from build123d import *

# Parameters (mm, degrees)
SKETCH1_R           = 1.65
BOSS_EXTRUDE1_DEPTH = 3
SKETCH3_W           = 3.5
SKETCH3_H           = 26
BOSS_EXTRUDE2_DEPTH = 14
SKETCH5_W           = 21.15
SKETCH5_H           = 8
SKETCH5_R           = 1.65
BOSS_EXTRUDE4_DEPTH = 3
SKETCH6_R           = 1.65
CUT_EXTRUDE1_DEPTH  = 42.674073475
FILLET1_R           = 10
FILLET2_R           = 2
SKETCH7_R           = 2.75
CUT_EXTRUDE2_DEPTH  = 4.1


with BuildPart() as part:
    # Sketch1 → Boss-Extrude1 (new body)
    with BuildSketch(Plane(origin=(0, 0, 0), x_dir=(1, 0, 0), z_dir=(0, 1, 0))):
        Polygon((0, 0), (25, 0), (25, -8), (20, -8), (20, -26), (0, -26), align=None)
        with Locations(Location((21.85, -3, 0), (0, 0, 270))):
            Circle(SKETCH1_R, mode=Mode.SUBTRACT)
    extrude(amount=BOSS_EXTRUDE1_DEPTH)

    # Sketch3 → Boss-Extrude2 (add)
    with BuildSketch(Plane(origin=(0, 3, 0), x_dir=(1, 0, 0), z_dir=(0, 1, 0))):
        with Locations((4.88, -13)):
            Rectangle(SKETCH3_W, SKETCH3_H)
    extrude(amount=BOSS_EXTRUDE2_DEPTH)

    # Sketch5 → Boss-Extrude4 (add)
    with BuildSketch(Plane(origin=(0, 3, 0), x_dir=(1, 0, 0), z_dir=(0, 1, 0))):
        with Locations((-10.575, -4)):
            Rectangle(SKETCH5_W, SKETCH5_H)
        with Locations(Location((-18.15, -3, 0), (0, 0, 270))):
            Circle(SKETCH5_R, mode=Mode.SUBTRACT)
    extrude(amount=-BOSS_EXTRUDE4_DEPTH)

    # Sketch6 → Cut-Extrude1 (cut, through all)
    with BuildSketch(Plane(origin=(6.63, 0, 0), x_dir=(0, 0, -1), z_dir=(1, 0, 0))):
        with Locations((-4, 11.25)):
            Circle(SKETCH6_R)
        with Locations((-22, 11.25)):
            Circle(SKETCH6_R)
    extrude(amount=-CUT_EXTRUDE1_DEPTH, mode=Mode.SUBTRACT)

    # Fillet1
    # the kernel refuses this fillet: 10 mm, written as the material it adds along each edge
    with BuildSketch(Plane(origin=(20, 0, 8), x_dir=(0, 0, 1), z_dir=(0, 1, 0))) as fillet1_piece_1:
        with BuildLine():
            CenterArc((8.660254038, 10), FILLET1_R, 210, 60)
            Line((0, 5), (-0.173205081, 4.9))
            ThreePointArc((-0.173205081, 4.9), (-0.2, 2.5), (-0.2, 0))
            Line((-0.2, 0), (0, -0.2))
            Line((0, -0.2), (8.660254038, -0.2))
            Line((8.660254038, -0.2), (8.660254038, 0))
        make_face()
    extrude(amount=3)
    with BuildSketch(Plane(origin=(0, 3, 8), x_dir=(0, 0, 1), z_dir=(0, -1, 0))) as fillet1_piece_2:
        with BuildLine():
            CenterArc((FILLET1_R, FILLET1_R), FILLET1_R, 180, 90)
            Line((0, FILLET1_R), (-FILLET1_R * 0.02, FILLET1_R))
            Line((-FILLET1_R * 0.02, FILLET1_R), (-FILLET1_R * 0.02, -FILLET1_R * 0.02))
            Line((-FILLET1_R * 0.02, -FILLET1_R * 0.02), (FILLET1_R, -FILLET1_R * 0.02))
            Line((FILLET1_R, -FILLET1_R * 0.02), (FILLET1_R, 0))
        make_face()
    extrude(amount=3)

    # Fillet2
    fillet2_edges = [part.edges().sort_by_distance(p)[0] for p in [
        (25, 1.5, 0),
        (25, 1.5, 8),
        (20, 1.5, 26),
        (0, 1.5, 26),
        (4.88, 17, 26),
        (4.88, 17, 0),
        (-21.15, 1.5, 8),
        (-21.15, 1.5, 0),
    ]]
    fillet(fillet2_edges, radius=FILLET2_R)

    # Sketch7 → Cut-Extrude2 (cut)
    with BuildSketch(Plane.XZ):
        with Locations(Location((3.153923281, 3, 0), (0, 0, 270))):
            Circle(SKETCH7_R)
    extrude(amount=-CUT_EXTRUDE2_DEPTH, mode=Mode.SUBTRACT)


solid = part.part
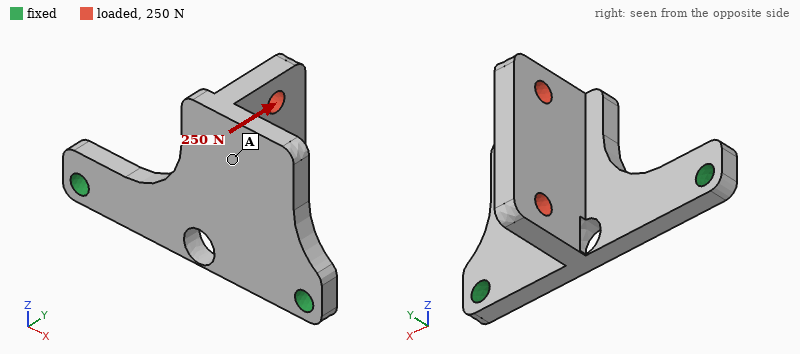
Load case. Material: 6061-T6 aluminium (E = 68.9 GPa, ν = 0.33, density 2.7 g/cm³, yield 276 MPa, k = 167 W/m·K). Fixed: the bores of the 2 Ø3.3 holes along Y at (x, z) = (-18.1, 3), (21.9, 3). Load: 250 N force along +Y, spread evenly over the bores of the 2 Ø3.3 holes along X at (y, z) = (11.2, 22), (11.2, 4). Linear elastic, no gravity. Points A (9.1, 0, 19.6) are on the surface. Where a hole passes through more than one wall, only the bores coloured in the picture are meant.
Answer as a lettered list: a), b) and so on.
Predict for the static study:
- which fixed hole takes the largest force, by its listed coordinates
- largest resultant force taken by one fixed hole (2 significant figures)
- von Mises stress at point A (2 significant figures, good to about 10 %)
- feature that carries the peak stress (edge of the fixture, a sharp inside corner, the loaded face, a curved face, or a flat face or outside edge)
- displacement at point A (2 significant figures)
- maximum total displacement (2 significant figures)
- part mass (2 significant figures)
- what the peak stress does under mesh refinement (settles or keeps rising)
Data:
a) (21.9, 3)
b) 150 N
c) 19 MPa
d) edge of the fixture
e) 0.12 mm
f) 0.21 mm
g) 9.0 g
h) keeps rising
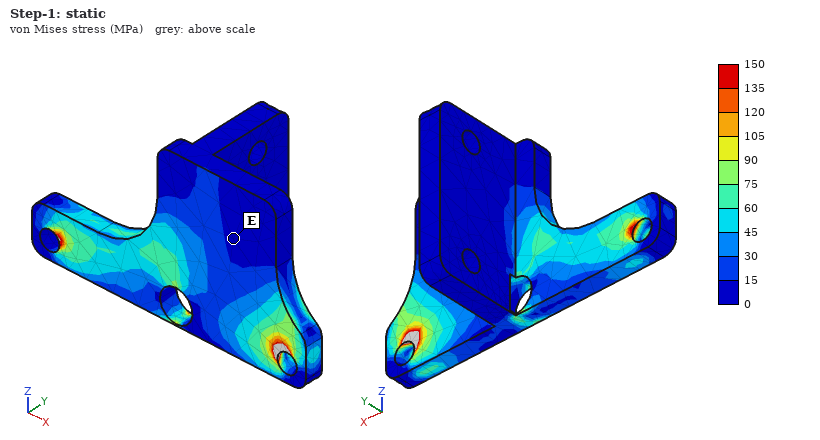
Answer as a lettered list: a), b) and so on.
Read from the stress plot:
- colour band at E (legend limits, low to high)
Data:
a) 0 to 15 MPa
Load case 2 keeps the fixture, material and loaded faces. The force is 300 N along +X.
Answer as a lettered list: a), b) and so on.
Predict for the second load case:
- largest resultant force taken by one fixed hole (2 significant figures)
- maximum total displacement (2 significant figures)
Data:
a) 190 N
b) 0.11 mm
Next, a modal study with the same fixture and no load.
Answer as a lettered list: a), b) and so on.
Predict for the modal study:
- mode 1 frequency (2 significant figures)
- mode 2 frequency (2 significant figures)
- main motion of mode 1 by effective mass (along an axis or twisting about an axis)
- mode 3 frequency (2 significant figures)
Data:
a) 2500 Hz
b) 5300 Hz
c) along Y
d) 7700 Hz
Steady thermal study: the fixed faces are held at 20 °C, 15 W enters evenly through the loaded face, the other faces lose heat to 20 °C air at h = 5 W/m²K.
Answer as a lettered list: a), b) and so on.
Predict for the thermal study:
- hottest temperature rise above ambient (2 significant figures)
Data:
a) 37 K
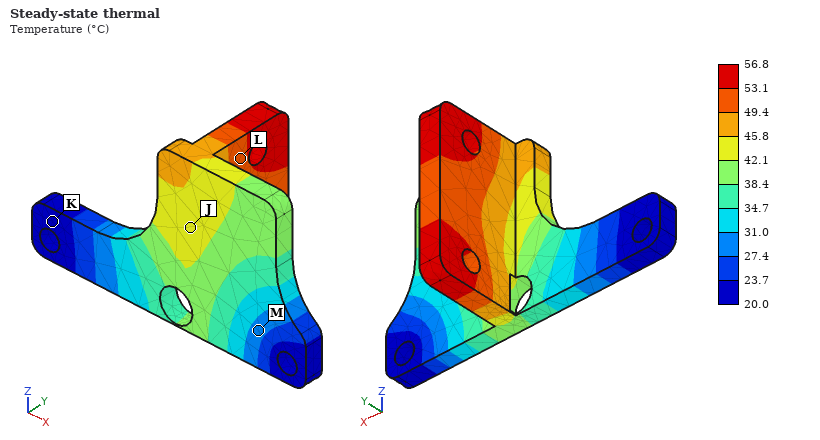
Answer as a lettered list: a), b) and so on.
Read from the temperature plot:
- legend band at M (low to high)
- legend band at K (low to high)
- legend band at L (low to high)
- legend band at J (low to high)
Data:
a) 27.4 to 31.0 °C
b) 20.0 to 23.7 °C
c) 49.4 to 53.1 °C
d) 42.1 to 45.8 °C
